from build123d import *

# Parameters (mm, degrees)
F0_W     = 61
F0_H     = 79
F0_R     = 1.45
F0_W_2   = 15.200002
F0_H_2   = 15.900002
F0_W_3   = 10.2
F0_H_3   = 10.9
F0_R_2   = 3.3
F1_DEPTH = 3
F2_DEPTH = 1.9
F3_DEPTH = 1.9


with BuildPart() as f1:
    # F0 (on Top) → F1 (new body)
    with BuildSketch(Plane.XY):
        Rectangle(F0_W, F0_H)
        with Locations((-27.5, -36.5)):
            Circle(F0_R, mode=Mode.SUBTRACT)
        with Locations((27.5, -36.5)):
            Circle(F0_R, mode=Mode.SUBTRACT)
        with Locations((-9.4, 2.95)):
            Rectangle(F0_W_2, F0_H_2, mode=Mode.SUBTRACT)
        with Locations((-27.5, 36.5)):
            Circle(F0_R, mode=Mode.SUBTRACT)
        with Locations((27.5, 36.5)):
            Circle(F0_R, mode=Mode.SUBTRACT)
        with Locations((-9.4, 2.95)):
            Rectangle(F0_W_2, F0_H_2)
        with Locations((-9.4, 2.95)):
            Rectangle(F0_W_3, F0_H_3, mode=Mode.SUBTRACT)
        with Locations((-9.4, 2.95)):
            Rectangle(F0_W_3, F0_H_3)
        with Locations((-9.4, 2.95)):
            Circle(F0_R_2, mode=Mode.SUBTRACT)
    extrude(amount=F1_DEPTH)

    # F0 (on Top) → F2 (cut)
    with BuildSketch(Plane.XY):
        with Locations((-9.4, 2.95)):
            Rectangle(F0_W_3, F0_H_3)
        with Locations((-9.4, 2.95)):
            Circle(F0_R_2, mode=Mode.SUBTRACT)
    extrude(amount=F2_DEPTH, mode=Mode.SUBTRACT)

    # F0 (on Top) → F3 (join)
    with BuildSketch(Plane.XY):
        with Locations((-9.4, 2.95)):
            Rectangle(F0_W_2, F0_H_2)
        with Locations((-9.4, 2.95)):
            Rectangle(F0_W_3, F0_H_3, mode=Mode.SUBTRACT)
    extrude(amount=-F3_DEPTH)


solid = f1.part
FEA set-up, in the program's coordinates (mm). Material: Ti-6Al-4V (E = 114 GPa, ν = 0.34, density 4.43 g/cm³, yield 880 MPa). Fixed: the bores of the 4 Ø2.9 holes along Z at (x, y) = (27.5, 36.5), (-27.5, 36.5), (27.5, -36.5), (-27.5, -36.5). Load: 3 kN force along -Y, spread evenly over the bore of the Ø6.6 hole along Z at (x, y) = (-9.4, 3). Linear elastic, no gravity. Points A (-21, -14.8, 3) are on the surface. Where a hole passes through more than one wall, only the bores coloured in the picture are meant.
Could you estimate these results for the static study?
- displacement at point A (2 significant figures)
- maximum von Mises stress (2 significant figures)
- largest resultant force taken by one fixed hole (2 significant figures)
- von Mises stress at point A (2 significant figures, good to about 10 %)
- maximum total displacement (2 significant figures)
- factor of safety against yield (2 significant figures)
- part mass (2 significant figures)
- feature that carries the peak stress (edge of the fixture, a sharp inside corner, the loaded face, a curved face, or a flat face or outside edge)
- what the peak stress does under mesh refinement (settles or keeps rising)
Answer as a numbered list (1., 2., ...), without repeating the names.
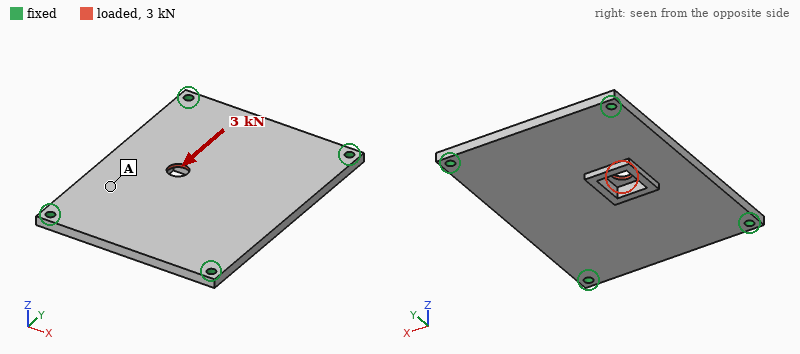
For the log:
1. 9.7 µm
2. 230 MPa
3. 1000 N
4. 24 MPa
5. 14 µm
6. 3.8
7. 64 g
8. the loaded face
9. settles
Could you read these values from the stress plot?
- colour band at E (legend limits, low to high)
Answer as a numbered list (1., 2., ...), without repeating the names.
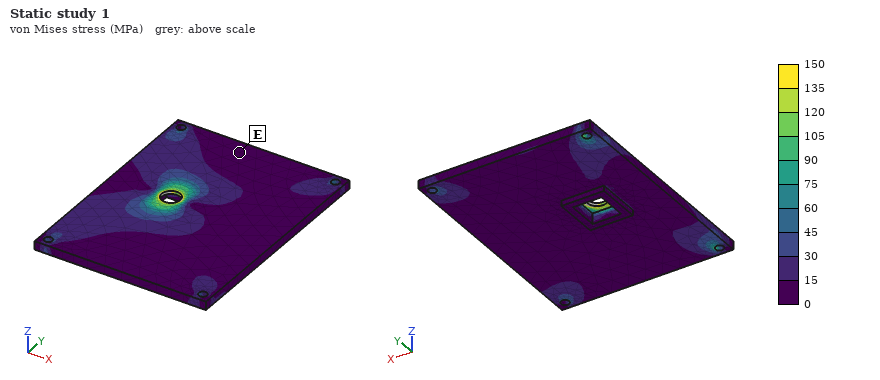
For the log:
1. 0 to 15 MPa
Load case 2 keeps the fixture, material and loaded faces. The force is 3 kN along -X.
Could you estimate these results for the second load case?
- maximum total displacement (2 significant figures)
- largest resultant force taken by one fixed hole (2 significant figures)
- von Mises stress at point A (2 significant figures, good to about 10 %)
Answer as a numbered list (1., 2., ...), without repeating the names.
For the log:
1. 30 µm
2. 970 N
3. 23 MPa
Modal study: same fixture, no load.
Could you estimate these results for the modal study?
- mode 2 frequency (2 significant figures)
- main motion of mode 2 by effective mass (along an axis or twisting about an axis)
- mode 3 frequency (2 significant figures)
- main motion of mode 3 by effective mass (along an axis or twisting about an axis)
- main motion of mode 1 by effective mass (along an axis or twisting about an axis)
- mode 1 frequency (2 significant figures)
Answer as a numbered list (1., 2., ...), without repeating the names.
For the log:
1. 3600 Hz
2. twisting about Y
3. 4800 Hz
4. twisting about X
5. along Z
6. 2200 Hz
